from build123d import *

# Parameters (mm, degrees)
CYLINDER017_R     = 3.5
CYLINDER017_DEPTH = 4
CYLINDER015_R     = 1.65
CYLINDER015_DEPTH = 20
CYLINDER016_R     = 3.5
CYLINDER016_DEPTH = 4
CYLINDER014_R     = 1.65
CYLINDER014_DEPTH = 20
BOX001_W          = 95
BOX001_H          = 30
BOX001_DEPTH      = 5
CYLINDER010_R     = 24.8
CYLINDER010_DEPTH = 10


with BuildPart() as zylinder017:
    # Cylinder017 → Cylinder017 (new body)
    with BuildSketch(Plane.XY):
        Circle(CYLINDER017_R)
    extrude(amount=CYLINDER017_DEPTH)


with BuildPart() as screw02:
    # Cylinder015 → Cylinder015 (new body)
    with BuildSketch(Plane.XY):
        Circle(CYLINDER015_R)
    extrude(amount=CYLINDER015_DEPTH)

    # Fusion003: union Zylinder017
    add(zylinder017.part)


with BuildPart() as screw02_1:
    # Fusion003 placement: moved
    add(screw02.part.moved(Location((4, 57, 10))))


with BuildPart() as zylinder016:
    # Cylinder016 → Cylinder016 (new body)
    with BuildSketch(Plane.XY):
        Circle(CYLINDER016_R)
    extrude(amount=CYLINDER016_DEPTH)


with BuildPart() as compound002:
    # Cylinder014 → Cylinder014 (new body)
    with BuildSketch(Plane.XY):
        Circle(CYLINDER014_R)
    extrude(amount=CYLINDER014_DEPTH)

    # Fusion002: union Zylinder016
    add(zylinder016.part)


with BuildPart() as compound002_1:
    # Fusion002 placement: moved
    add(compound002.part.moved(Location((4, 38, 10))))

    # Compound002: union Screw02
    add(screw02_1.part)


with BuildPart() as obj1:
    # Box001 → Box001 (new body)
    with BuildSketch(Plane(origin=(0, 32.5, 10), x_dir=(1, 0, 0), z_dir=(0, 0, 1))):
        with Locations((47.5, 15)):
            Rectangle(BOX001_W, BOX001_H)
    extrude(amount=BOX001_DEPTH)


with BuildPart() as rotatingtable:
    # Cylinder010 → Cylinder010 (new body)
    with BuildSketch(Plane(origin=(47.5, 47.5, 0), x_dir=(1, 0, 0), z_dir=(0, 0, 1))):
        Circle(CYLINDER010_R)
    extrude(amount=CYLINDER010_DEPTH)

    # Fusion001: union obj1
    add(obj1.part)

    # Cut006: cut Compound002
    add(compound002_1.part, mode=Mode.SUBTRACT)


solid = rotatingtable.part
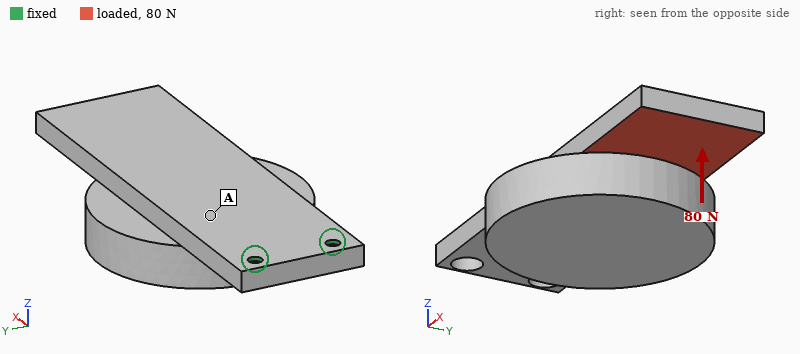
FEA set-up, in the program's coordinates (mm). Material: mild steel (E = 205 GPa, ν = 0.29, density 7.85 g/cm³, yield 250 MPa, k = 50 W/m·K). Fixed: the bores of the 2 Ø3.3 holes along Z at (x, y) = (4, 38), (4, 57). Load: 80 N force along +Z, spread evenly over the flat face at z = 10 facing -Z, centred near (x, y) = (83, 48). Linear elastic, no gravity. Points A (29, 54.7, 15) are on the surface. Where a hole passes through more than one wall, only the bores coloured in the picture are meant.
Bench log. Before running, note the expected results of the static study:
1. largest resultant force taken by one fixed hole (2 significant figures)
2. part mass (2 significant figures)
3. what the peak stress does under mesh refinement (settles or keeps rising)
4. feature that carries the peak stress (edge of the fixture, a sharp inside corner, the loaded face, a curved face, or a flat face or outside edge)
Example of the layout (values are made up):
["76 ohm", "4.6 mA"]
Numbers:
["53 N", "260 g", "keeps rising", "edge of the fixture"]
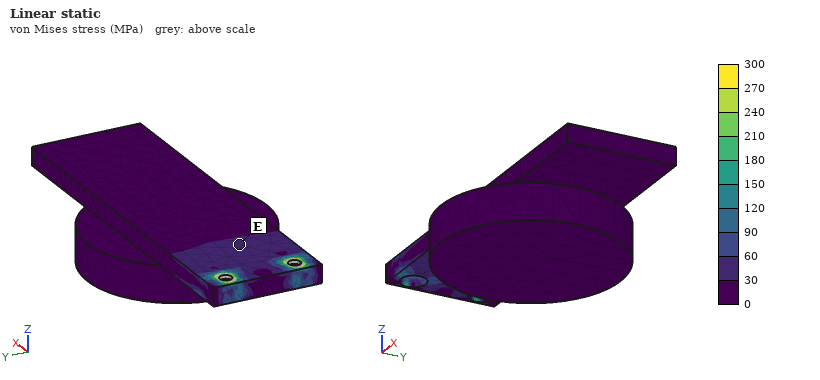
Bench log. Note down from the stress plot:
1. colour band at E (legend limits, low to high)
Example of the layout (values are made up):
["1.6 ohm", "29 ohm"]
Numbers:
["30 to 60 MPa"]
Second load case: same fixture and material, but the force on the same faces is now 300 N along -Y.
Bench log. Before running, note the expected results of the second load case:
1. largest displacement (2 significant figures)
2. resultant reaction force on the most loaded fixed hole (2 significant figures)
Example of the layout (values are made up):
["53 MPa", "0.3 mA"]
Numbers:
["48 µm", "1.2 kN"]
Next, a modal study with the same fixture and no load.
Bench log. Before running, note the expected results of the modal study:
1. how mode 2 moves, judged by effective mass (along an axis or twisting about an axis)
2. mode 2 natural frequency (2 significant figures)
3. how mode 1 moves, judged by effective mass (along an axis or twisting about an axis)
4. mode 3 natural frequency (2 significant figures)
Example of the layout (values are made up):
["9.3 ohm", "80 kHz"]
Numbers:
["along Y", "1500 Hz", "along Z", "1800 Hz"]
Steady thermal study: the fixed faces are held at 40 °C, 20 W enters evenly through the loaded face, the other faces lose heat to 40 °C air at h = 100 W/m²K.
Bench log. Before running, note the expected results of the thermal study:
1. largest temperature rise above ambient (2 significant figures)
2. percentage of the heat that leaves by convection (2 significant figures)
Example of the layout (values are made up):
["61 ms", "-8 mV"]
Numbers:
["55 K", "88 %"]
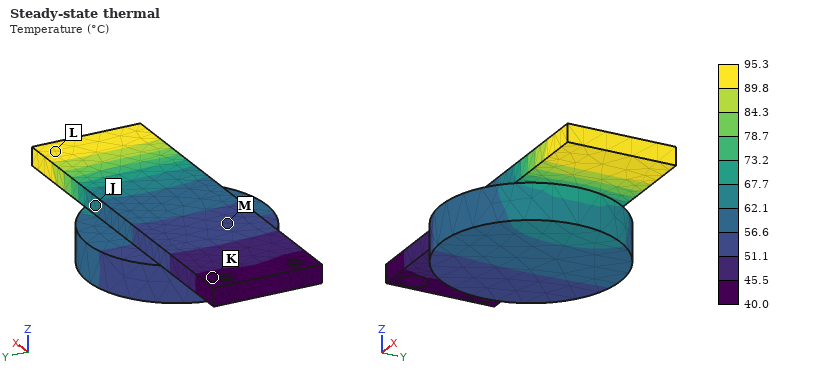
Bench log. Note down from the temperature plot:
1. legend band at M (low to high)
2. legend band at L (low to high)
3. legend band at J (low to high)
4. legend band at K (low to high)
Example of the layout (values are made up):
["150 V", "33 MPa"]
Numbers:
["51.1 to 56.6 °C", "89.8 to 95.3 °C", "62.1 to 67.7 °C", "40.0 to 45.5 °C"]
